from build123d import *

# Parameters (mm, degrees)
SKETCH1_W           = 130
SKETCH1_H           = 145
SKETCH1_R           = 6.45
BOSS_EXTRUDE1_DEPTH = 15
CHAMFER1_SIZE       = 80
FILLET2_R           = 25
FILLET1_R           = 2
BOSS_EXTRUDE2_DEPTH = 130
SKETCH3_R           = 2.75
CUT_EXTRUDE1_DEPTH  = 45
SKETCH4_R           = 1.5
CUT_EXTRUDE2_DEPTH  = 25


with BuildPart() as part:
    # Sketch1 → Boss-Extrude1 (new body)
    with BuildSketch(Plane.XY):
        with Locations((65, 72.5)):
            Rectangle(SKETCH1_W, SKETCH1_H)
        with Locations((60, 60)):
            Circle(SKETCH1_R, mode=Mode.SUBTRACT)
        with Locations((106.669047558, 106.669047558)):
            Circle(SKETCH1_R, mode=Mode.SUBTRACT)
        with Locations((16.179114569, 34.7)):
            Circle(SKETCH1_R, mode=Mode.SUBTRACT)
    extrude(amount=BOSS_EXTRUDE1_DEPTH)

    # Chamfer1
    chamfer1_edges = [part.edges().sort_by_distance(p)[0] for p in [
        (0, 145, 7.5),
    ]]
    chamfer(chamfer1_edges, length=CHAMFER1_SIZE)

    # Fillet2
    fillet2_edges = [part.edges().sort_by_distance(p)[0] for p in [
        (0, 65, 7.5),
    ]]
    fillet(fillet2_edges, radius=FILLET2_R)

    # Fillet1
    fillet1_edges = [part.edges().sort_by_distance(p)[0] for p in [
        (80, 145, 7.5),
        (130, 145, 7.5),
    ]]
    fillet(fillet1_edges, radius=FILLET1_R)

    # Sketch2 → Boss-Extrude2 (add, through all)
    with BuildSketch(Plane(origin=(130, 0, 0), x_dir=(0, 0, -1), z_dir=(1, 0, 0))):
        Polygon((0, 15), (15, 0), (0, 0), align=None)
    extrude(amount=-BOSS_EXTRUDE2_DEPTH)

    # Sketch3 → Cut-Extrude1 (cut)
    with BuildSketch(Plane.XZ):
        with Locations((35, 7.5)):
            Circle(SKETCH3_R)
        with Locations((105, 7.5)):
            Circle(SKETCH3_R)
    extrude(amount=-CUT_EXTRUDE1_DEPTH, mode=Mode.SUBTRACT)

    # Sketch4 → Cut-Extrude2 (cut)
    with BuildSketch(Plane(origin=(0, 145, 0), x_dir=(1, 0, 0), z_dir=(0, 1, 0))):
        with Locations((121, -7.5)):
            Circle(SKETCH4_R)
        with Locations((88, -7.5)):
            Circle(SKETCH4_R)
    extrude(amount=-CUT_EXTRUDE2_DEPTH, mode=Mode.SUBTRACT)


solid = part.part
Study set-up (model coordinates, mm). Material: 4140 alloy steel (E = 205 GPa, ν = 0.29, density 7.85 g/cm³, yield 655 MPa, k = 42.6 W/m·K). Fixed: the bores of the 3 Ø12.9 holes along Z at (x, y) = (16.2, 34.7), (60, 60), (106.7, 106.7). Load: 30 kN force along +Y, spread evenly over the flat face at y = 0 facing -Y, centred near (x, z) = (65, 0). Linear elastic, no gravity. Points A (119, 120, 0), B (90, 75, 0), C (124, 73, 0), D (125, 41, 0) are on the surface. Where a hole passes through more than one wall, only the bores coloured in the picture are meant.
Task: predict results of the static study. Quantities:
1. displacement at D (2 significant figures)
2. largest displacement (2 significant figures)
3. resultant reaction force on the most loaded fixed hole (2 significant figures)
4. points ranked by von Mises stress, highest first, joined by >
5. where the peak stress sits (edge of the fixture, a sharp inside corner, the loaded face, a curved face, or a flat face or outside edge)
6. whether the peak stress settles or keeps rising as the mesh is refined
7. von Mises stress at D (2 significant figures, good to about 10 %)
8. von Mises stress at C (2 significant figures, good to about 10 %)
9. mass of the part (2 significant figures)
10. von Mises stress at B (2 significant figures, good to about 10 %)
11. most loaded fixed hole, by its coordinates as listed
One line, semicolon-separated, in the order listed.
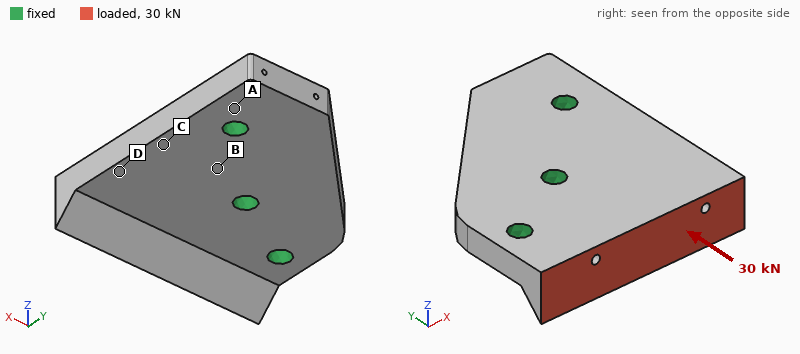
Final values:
16 µm; 77 µm; 12 kN; D > C > B > A; edge of the fixture; keeps rising; 46 MPa; 30 MPa; 1.9 kg; 21 MPa; (60, 60)
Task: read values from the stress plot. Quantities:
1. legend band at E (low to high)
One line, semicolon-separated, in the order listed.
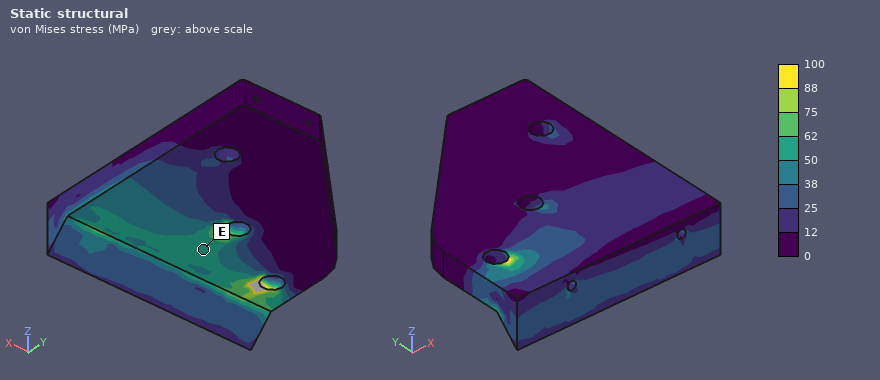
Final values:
50 to 62 MPa
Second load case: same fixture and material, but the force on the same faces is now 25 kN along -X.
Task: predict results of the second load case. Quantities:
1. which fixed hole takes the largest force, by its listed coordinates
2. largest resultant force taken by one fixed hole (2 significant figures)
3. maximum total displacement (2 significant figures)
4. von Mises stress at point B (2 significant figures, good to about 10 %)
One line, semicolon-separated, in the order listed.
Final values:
(16.2, 34.7); 20 kN; 54 µm; 13 MPa
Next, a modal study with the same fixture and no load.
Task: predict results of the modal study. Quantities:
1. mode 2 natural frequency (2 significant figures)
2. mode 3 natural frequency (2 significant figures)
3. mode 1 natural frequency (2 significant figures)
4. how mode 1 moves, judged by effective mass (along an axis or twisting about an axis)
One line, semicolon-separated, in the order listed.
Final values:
5800 Hz; 6000 Hz; 2300 Hz; along Z
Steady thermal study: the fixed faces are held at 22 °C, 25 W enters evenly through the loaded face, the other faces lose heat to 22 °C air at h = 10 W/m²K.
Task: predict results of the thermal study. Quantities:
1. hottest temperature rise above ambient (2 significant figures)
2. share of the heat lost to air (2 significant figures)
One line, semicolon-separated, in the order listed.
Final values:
21 K; 7.7 %
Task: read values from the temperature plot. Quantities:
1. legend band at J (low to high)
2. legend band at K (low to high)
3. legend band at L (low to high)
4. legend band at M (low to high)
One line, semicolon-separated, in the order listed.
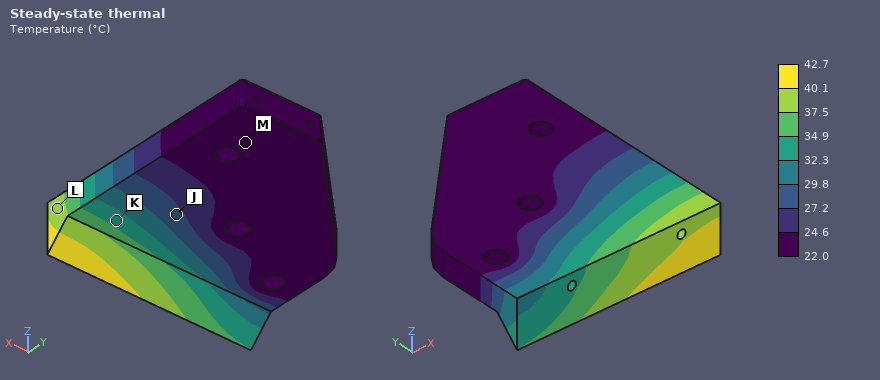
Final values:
27.2 to 29.8 °C; 32.3 to 34.9 °C; 37.5 to 40.1 °C; 22.0 to 24.6 °C
